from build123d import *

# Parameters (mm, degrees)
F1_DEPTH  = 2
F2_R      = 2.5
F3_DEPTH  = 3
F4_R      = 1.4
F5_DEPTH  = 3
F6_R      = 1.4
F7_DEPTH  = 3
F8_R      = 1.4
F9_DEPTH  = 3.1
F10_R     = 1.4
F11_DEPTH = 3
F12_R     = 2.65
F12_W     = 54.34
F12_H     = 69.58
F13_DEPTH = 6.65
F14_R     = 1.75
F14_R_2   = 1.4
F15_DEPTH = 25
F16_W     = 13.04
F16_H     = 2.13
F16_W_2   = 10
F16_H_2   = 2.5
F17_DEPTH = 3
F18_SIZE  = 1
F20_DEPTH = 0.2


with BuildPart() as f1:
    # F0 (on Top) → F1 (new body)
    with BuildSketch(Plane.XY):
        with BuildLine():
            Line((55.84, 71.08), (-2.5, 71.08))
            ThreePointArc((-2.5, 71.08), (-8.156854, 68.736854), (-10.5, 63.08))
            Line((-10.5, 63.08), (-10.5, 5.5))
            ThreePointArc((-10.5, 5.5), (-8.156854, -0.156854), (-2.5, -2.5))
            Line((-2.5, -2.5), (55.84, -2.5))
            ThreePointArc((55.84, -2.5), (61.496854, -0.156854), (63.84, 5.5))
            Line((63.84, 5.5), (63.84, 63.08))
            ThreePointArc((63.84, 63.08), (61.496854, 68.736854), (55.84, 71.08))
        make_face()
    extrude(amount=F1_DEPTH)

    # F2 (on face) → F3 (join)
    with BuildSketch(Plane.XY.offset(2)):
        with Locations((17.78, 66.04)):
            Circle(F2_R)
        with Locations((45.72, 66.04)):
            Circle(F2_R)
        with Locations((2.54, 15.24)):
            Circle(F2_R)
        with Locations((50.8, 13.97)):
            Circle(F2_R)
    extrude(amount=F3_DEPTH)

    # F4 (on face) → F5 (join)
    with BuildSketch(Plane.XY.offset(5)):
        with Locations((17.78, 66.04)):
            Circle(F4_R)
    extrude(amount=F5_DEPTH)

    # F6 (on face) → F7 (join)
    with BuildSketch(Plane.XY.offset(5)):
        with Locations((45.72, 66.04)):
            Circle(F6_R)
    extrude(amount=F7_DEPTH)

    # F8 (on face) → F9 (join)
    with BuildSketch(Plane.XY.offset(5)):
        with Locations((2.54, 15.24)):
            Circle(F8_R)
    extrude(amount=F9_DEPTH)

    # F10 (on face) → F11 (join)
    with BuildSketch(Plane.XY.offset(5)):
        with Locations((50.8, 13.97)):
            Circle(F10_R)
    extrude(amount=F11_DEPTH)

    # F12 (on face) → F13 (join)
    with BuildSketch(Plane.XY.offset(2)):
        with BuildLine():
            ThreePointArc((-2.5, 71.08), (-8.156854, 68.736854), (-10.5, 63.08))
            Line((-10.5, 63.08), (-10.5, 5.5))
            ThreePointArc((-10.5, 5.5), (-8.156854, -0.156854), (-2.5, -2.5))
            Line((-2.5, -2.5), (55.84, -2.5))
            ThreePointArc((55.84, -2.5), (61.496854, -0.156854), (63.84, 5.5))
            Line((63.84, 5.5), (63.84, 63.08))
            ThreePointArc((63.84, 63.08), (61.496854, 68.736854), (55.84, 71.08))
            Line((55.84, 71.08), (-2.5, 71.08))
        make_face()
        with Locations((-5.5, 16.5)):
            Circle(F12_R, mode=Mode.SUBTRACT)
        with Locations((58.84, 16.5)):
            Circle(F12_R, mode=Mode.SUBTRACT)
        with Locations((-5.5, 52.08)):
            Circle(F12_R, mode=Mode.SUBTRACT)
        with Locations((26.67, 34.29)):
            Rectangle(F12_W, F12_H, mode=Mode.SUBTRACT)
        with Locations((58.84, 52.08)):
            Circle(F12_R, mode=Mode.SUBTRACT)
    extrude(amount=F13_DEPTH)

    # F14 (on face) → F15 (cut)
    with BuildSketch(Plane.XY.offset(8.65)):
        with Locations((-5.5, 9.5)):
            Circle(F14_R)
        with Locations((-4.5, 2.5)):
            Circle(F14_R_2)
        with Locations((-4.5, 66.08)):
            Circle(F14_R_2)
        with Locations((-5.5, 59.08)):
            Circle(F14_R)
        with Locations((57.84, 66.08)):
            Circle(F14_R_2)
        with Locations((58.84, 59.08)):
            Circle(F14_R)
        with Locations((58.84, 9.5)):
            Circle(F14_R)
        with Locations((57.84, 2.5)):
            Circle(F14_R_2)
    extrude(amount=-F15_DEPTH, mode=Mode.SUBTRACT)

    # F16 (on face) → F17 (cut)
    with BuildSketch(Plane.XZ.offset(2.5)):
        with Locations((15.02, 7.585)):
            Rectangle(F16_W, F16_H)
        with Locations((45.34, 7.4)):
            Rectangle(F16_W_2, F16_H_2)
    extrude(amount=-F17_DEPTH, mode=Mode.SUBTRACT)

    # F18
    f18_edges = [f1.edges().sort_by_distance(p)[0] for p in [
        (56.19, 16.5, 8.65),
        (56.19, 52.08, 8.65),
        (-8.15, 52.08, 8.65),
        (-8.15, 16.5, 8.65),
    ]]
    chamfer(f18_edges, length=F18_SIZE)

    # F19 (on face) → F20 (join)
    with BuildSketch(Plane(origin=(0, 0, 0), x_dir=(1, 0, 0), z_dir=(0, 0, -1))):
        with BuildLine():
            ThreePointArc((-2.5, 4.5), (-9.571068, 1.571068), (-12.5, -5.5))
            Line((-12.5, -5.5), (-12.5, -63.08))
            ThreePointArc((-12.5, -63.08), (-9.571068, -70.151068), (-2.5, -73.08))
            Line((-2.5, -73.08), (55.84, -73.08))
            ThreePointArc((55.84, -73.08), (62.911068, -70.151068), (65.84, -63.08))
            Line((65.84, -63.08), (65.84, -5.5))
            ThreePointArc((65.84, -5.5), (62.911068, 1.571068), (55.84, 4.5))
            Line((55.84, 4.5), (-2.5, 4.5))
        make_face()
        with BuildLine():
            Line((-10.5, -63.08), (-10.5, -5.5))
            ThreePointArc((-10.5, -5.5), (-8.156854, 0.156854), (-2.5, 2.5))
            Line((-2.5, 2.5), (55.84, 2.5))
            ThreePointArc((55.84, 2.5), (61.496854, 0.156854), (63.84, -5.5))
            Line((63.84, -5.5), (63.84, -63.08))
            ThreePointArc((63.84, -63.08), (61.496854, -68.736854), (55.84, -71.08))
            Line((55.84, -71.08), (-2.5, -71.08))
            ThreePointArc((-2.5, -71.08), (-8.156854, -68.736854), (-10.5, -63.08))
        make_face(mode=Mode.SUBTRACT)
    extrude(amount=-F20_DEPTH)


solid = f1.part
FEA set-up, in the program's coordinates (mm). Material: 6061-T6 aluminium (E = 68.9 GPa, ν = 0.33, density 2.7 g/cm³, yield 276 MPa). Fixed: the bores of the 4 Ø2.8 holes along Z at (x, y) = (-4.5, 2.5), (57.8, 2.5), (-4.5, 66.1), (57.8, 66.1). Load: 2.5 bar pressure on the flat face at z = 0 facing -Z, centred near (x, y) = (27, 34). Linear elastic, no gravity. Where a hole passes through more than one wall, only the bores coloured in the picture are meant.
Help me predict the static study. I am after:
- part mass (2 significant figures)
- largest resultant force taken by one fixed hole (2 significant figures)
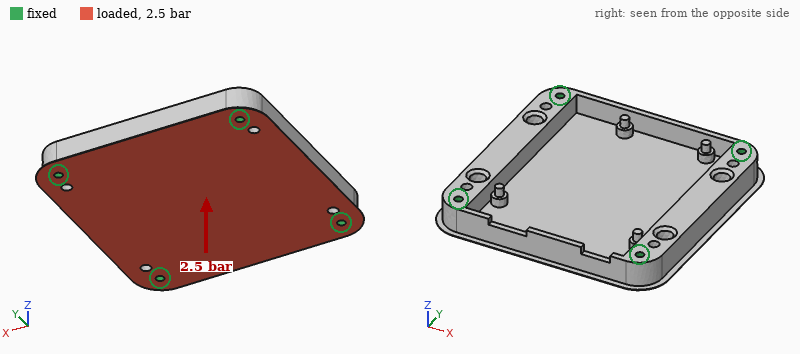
56 g
430 N
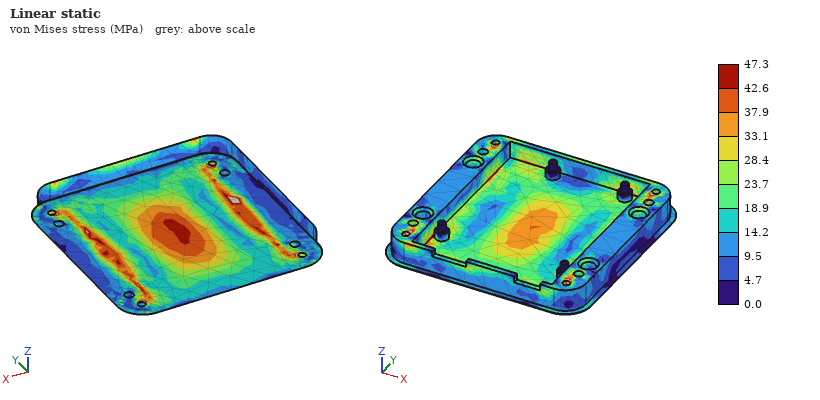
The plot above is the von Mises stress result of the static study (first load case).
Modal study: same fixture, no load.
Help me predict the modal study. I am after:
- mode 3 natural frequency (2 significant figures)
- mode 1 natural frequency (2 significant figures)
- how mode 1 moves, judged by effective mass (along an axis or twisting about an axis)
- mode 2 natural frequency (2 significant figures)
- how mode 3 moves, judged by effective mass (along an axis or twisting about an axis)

7600 Hz
3700 Hz
along Z
5900 Hz
twisting about Y
